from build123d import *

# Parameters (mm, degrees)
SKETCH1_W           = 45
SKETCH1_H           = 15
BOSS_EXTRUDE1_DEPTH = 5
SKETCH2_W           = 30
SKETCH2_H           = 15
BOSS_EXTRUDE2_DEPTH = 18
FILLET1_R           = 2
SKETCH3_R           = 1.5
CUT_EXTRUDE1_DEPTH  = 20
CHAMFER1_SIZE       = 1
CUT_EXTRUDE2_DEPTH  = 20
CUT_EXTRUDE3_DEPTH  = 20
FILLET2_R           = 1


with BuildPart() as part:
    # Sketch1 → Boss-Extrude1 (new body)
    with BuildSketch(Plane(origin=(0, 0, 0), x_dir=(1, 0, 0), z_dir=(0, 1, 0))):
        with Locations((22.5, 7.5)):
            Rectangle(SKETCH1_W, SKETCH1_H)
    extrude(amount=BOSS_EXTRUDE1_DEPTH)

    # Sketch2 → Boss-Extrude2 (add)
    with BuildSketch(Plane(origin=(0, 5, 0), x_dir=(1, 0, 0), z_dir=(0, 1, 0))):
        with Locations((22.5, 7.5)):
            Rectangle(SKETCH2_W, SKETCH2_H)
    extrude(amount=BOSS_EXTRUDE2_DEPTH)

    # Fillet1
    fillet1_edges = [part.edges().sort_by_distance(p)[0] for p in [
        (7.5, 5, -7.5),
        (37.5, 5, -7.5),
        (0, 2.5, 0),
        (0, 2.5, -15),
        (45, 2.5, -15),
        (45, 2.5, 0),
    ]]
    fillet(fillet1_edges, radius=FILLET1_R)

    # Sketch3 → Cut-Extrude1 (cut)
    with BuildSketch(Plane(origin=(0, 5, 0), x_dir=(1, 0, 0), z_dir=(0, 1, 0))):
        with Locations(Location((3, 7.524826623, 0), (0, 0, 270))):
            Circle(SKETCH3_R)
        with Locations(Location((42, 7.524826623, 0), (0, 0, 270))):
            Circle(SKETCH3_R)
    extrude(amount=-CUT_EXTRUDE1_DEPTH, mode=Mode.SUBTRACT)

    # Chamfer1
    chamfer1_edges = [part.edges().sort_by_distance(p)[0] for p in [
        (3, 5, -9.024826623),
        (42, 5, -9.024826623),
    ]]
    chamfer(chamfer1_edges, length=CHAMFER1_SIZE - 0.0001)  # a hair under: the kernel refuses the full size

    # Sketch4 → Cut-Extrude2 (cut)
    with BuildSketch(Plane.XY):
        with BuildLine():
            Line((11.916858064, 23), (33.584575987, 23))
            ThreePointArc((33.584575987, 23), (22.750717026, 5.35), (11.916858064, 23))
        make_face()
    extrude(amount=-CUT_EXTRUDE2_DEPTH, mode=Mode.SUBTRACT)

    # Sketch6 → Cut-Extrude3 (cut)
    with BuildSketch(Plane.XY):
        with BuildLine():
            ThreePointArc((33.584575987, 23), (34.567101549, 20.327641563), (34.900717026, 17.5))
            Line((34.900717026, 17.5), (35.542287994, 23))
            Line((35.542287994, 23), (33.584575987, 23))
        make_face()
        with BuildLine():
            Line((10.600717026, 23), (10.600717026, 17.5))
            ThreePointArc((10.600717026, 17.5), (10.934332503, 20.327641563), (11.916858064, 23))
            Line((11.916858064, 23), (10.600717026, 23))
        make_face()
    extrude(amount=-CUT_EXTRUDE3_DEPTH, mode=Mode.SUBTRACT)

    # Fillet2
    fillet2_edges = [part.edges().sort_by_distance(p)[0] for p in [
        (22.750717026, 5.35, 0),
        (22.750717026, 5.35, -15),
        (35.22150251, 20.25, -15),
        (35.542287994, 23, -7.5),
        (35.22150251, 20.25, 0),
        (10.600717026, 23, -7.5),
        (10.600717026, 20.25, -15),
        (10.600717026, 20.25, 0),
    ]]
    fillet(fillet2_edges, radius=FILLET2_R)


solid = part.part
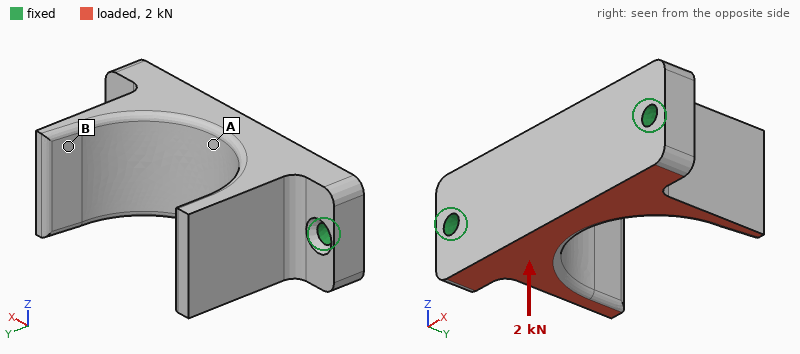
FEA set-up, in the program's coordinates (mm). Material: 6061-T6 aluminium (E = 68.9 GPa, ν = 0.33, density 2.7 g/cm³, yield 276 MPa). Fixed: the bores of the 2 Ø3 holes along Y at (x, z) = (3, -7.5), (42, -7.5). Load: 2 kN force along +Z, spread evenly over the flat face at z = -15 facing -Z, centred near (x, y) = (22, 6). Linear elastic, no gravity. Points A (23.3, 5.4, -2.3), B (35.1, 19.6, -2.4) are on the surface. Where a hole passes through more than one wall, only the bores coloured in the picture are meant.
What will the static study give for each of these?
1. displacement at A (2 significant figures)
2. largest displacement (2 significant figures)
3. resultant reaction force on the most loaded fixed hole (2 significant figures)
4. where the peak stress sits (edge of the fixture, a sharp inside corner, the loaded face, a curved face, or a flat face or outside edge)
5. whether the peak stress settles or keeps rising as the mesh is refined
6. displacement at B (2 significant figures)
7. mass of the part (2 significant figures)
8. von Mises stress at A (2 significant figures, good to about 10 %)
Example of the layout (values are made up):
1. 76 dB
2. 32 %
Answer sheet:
1. 19 µm
2. 52 µm
3. 1.0 kN
4. edge of the fixture
5. keeps rising
6. 40 µm
7. 16 g
8. 27 MPa
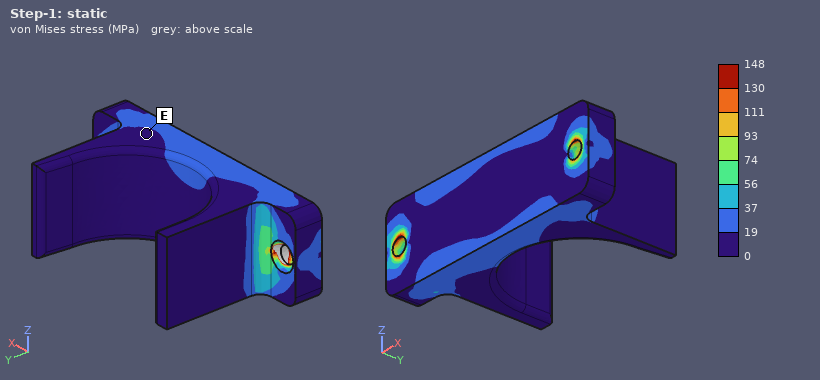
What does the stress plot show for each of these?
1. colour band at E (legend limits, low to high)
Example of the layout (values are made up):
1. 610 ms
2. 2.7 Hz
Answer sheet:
1. 0 to 19 MPa
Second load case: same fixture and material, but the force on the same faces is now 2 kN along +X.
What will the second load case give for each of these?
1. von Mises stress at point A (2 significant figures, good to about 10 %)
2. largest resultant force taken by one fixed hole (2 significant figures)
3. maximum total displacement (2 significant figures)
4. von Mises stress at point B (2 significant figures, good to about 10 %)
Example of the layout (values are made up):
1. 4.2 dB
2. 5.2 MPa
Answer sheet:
1. 6.0 MPa
2. 1.1 kN
3. 35 µm
4. 7.3 MPa
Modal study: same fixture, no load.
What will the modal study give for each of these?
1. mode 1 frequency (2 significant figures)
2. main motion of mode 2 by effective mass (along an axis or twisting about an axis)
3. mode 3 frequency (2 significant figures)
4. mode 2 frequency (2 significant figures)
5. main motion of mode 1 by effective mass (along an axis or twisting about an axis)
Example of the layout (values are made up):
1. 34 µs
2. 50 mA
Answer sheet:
1. 9100 Hz
2. along Y
3. 15 kHz
4. 9600 Hz
5. along Z
